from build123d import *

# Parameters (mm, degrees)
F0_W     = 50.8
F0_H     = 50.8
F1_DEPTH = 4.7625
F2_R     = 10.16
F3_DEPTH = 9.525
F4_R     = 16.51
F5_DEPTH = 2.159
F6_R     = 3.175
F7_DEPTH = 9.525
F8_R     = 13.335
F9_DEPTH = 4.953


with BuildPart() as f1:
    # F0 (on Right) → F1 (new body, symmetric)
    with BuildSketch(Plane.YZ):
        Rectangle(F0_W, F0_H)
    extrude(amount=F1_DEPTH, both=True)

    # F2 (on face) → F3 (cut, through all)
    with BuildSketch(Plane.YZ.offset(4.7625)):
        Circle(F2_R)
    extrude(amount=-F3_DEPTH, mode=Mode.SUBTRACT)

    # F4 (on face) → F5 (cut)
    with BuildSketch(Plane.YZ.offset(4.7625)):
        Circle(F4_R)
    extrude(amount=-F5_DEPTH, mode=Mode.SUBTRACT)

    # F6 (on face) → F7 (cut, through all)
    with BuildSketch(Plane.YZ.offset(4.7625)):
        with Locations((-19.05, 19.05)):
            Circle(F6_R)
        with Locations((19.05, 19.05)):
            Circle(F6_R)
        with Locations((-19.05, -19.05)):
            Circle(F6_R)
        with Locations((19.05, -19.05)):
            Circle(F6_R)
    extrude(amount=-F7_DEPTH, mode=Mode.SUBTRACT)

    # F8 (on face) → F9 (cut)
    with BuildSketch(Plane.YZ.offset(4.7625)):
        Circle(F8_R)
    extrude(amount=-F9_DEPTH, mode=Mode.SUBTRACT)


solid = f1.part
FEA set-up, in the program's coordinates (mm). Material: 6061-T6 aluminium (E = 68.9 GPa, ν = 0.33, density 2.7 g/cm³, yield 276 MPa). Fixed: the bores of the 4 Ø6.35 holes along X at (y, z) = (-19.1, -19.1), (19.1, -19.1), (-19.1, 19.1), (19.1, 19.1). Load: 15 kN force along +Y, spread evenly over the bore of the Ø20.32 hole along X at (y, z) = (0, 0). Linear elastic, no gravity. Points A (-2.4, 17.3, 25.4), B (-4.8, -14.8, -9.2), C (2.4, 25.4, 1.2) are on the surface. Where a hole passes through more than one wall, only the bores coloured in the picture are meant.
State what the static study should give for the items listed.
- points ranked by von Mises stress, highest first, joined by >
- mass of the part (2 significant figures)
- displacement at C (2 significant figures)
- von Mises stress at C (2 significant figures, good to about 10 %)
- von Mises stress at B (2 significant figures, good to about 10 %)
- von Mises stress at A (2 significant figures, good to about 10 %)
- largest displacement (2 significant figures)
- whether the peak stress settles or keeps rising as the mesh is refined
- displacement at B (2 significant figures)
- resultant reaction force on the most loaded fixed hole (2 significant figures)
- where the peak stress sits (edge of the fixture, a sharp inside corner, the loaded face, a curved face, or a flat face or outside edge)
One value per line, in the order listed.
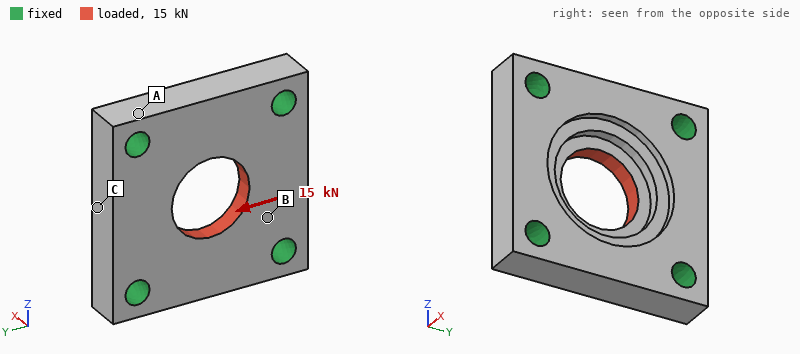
B > C > A
50 g
9.5 µm
30 MPa
55 MPa
10 MPa
21 µm
keeps rising
9.6 µm
4.0 kN
edge of the fixture
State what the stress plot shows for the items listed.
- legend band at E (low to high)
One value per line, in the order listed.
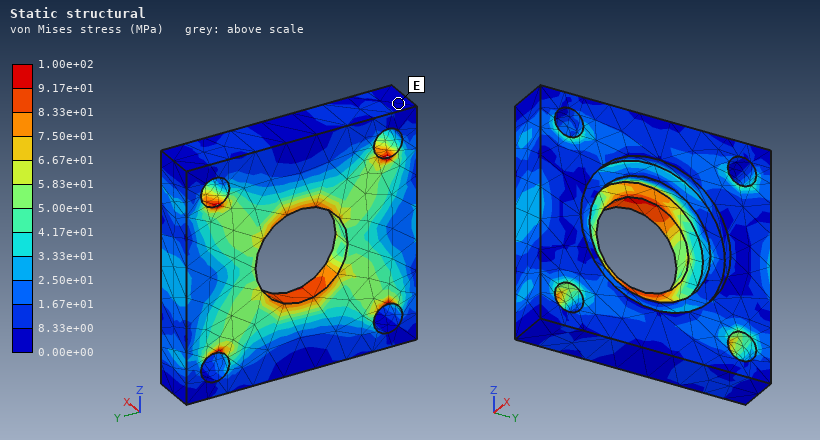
0.00e+00 to 8.33e+00 MPa
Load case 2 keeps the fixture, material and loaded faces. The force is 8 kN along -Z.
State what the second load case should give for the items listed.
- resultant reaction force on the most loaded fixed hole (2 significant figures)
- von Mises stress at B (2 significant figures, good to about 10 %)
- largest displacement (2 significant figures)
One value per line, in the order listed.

2.1 kN
19 MPa
11 µm
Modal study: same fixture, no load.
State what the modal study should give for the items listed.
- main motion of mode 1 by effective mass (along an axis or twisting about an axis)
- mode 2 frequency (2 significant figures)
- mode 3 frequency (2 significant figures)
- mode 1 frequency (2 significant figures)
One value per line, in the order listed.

along X
29 kHz
30 kHz
26 kHz
